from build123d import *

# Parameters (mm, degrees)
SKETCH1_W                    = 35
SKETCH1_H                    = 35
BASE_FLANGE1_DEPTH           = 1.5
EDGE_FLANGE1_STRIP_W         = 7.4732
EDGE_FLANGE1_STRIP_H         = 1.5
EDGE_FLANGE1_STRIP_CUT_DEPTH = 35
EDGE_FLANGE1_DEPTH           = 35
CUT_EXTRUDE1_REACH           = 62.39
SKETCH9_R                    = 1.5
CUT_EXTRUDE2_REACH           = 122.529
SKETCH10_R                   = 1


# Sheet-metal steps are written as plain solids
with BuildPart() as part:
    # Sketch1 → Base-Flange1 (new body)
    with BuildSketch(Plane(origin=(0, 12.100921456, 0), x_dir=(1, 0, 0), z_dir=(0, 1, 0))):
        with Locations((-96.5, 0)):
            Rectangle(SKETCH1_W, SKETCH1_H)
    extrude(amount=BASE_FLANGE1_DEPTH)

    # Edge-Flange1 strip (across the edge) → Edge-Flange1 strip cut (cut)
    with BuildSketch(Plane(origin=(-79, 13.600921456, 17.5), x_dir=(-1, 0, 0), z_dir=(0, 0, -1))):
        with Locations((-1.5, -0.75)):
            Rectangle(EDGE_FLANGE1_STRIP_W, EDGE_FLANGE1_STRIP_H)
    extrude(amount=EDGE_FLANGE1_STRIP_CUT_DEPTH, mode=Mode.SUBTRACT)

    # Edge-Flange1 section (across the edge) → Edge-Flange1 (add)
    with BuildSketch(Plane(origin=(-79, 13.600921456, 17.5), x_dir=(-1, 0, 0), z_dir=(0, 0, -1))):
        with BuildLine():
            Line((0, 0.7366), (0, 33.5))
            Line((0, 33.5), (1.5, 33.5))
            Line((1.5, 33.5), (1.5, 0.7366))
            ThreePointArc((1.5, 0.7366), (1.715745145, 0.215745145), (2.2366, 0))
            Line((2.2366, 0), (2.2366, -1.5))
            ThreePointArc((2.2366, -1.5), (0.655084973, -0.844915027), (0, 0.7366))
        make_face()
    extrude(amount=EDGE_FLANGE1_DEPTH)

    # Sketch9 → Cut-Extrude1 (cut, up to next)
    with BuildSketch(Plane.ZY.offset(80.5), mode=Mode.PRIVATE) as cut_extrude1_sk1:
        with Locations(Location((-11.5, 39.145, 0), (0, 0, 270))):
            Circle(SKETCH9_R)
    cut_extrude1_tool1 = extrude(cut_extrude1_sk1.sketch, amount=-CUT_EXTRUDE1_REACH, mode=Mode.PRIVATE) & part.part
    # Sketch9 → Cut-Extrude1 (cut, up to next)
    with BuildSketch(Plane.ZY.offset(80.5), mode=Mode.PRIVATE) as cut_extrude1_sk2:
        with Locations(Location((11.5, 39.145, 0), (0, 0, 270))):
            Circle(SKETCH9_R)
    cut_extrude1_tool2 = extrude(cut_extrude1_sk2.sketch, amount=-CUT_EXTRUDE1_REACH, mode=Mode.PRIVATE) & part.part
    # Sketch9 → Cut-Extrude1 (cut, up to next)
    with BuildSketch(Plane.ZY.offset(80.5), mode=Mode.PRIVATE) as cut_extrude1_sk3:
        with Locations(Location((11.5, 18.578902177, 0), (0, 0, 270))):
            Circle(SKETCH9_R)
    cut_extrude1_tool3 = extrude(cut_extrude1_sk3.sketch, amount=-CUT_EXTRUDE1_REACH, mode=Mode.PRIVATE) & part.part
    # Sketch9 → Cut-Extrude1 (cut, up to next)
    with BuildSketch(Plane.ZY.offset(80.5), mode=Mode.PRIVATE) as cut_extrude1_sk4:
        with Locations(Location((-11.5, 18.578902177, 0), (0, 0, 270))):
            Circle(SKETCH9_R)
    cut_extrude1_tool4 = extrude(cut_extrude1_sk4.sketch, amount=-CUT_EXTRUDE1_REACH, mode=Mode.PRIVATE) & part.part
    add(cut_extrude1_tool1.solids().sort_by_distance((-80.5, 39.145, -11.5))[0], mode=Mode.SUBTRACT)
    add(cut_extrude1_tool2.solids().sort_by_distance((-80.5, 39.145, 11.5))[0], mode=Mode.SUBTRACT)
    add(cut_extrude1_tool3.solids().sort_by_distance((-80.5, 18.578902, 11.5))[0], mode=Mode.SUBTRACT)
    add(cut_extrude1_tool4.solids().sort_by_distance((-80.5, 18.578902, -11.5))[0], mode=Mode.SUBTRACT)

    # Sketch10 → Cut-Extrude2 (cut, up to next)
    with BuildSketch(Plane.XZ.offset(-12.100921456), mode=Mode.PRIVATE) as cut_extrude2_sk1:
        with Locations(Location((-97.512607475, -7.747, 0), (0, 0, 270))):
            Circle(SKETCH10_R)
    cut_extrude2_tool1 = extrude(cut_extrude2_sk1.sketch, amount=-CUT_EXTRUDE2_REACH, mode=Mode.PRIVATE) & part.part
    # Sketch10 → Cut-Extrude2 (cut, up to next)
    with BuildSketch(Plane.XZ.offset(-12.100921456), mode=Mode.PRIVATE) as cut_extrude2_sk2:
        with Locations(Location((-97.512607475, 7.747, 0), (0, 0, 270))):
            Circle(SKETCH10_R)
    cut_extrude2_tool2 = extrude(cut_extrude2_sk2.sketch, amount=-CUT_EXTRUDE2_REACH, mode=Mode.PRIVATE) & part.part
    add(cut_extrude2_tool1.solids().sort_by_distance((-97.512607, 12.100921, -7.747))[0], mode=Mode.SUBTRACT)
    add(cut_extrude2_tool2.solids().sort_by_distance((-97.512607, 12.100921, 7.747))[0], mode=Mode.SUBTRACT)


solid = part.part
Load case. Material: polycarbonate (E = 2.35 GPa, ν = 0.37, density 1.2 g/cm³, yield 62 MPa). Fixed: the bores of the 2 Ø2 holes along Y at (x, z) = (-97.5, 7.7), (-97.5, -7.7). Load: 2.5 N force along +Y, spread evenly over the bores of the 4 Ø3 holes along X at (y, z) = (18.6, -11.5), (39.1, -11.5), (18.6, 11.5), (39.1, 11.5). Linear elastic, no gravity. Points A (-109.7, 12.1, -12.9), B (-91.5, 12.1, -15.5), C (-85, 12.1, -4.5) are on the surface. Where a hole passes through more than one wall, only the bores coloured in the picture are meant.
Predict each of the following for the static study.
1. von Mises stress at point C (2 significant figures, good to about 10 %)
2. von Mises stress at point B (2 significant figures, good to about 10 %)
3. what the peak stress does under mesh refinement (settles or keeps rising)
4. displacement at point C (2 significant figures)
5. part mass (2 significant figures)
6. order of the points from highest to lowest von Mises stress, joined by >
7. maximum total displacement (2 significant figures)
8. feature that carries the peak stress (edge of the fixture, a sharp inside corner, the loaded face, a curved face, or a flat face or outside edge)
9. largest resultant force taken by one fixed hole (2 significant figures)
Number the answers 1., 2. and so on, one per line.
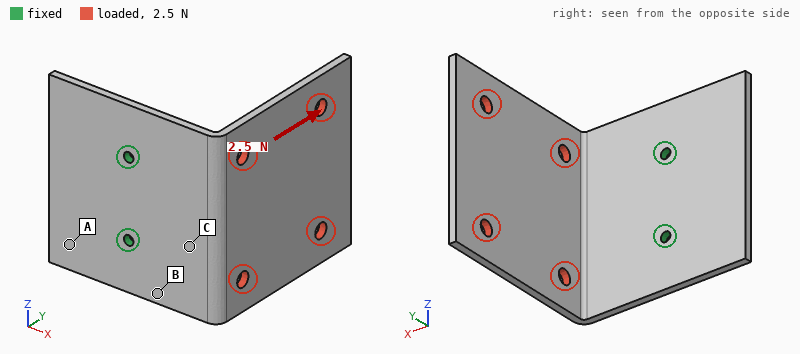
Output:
1. 0.89 MPa
2. 1.9 MPa
3. keeps rising
4. 0.13 mm
5. 4.2 g
6. B > C > A
7. 0.63 mm
8. edge of the fixture
9. 1.3 N
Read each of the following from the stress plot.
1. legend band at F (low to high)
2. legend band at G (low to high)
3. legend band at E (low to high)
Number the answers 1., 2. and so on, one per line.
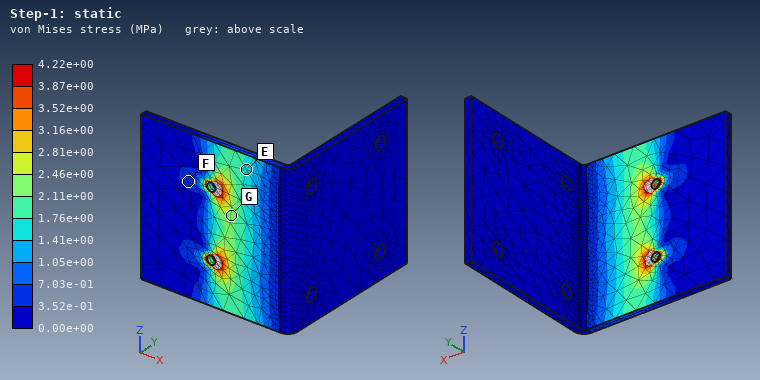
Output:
1. 3.52e-01 to 7.03e-01 MPa
2. 2.11e+00 to 2.46e+00 MPa
3. 1.41e+00 to 1.76e+00 MPa
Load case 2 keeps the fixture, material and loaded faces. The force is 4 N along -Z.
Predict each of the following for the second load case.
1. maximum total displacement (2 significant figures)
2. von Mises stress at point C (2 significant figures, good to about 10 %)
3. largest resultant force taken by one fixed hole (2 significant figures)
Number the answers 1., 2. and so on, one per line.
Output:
1. 0.66 mm
2. 2.3 MPa
3. 5.7 N
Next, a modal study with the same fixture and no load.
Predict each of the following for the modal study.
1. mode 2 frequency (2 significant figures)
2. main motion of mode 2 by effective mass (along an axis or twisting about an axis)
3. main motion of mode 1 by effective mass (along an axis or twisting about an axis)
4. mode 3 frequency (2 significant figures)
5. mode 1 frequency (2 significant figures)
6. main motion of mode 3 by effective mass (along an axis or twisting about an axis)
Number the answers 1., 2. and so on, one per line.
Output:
1. 300 Hz
2. along Z
3. along X
4. 530 Hz
5. 160 Hz
6. along Y
